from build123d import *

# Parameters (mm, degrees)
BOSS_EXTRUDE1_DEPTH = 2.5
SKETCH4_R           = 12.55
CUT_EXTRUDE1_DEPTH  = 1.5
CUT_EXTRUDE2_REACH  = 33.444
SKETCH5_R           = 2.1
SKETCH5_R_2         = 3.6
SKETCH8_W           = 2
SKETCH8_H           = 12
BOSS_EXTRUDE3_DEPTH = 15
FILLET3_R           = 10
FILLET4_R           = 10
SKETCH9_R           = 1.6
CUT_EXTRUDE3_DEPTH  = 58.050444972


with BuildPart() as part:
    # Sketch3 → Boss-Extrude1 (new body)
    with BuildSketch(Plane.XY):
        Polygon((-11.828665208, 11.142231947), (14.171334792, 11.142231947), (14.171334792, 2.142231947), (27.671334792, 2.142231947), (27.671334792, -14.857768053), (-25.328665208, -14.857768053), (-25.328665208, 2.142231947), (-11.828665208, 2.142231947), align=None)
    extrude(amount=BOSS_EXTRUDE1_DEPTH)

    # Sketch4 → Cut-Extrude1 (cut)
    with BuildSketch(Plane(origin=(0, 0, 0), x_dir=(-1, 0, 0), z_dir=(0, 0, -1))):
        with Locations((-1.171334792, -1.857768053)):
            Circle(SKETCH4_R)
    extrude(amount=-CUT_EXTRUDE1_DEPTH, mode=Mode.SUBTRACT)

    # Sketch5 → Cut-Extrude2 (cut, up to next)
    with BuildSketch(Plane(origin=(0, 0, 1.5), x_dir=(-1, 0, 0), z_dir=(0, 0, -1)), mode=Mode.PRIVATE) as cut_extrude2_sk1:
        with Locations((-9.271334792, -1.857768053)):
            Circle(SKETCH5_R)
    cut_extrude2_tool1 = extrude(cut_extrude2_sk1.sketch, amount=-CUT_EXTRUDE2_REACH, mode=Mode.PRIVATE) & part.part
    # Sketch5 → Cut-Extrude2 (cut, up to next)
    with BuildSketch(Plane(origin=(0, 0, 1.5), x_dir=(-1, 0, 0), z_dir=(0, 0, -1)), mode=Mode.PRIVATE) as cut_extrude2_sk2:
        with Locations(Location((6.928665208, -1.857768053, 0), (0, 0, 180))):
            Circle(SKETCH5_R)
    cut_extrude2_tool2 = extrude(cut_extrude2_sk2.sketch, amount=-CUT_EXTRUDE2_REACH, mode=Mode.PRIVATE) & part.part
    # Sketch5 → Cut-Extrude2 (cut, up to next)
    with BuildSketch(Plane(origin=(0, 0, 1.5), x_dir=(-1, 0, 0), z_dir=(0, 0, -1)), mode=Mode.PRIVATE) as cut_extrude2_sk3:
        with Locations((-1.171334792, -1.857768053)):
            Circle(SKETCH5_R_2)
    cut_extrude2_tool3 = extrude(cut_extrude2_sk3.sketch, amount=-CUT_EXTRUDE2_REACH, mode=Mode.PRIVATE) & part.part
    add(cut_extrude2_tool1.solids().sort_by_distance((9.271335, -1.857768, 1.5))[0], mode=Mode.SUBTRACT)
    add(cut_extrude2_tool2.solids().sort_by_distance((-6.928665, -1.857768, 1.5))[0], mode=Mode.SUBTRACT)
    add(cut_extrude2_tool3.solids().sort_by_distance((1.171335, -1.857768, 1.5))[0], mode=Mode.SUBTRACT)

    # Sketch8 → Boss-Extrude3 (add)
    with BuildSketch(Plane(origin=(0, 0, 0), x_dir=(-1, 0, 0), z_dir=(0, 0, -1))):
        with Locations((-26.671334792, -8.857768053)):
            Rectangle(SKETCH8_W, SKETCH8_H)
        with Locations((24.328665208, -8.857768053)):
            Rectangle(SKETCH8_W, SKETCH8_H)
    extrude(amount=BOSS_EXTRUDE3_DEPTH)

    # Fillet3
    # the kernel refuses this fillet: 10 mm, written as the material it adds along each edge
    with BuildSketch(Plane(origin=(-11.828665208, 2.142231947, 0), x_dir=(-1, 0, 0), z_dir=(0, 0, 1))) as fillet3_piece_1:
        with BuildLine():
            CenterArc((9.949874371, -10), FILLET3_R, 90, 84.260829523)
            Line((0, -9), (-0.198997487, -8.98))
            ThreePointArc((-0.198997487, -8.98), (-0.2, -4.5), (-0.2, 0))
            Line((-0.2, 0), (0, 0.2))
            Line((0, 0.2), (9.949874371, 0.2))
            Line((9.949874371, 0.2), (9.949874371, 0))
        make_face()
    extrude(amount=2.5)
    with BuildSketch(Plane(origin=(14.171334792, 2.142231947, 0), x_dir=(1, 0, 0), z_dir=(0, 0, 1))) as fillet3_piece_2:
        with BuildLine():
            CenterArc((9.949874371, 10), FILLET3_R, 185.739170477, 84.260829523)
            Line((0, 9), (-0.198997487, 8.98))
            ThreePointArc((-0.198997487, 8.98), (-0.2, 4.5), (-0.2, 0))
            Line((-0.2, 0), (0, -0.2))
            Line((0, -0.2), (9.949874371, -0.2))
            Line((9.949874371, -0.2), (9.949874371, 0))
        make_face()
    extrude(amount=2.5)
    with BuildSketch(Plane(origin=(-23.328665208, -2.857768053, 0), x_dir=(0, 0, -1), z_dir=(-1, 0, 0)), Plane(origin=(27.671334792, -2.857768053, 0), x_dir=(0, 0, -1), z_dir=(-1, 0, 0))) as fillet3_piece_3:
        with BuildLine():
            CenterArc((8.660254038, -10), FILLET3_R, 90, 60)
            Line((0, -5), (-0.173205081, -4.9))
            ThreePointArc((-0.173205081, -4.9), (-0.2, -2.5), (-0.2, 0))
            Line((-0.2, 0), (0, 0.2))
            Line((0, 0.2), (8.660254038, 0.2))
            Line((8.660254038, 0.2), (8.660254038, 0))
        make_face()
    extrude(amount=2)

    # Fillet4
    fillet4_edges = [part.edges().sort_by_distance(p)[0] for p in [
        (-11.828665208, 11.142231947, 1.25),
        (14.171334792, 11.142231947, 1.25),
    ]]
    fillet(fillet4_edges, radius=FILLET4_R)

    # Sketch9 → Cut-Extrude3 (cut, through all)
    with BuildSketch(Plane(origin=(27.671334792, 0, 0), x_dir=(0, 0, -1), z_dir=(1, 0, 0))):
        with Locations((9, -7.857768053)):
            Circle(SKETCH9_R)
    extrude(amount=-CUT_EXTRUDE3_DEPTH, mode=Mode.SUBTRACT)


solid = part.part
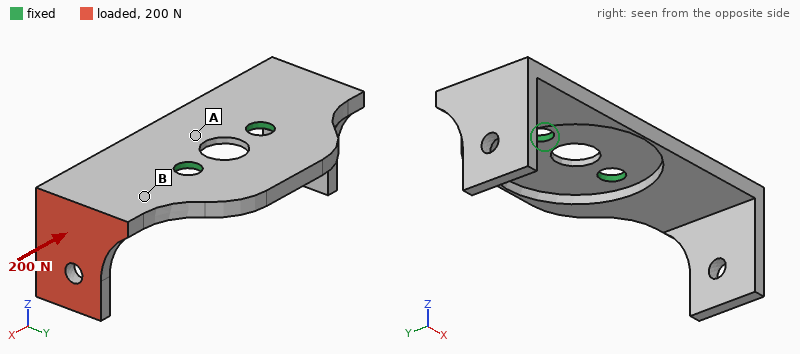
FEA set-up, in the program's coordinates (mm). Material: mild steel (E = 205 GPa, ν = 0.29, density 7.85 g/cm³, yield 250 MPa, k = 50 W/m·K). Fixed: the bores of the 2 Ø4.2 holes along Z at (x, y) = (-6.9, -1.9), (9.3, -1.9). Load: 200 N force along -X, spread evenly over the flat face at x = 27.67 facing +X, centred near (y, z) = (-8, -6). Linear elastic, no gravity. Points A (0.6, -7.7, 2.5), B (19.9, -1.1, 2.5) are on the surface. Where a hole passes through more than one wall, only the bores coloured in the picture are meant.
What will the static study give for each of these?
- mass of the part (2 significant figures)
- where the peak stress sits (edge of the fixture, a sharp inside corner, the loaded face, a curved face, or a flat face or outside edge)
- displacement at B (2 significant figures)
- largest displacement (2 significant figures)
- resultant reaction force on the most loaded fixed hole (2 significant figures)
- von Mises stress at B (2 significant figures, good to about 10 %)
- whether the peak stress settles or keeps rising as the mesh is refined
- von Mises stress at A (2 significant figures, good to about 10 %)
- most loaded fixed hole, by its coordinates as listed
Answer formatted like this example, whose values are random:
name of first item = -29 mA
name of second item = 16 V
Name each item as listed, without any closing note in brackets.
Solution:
mass of the part = 22 g
where the peak stress sits = edge of the fixture
displacement at B = 0.051 mm
largest displacement = 0.24 mm
resultant reaction force on the most loaded fixed hole = 160 N
von Mises stress at B = 65 MPa
whether the peak stress settles or keeps rising as the mesh is refined = keeps rising
von Mises stress at A = 25 MPa
most loaded fixed hole, by its coordinates as listed = (-6.9, -1.9)
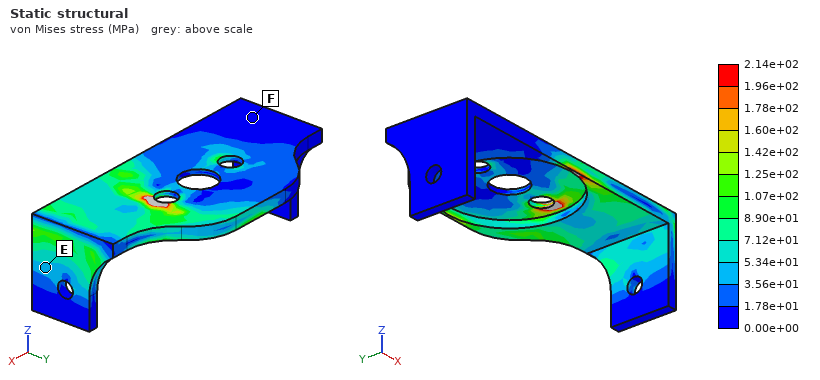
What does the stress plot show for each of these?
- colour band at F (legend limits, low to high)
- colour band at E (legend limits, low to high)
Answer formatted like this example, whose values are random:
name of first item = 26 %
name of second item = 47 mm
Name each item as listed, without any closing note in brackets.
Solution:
colour band at F = 0.00e+00 to 1.78e+01 MPa
colour band at E = 3.56e+01 to 5.34e+01 MPa
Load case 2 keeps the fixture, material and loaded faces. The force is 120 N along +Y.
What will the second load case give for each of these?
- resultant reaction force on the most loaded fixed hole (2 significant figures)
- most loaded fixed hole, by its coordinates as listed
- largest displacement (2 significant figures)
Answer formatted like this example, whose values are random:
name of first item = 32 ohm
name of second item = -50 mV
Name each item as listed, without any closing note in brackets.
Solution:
resultant reaction force on the most loaded fixed hole = 210 N
most loaded fixed hole, by its coordinates as listed = (9.3, -1.9)
largest displacement = 93 µm
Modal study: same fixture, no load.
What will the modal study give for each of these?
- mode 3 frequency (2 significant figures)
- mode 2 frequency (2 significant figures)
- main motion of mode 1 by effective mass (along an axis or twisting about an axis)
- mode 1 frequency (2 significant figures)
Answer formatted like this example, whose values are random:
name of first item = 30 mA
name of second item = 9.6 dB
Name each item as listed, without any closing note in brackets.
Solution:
mode 3 frequency = 3100 Hz
mode 2 frequency = 1800 Hz
main motion of mode 1 by effective mass = along Z
mode 1 frequency = 1700 Hz
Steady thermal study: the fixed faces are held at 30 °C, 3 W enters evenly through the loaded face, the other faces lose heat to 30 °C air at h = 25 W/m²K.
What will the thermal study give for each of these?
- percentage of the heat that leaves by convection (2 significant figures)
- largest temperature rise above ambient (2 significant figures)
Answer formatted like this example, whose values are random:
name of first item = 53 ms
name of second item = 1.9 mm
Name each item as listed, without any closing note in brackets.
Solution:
percentage of the heat that leaves by convection = 22 %
largest temperature rise above ambient = 40 K
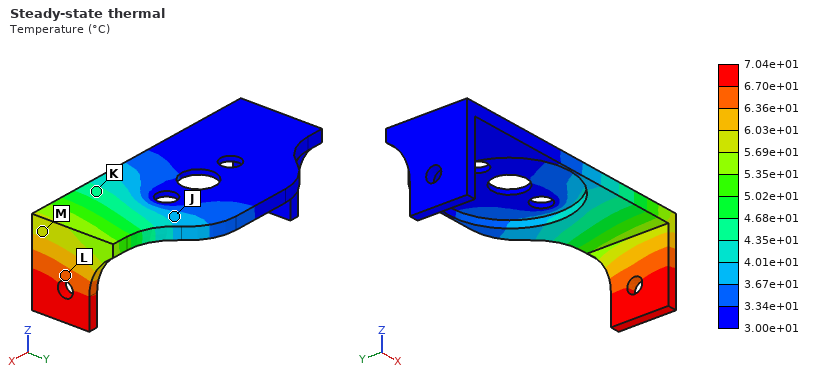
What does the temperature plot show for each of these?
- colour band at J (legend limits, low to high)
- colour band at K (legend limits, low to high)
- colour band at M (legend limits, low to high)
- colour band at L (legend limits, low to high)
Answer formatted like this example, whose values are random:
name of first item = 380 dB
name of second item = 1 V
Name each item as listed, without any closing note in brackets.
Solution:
colour band at J = 3.67e+01 to 4.01e+01 °C
colour band at K = 4.35e+01 to 4.68e+01 °C
colour band at M = 5.69e+01 to 6.03e+01 °C
colour band at L = 6.36e+01 to 6.70e+01 °C
